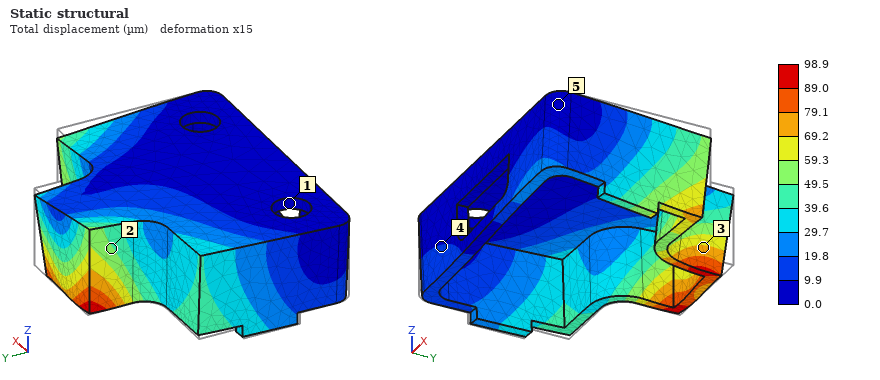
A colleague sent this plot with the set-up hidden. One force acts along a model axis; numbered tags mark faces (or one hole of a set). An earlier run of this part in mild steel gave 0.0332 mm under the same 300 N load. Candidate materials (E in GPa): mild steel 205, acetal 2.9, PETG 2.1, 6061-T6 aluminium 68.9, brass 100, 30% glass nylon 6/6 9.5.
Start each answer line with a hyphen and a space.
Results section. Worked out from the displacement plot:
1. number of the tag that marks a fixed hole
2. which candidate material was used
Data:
- 1
- 6061-T6 aluminium
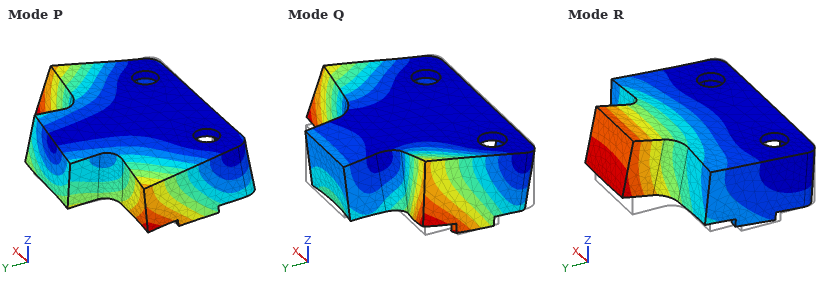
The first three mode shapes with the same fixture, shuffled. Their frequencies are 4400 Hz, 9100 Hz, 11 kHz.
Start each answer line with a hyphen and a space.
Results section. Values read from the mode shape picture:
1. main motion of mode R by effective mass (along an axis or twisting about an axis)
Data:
- along Z
